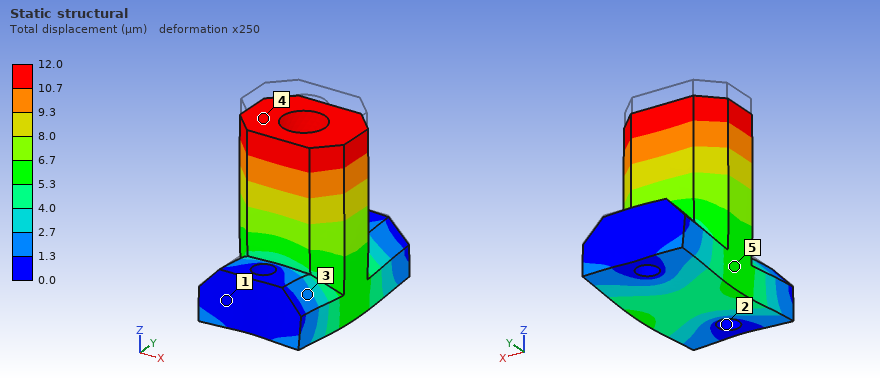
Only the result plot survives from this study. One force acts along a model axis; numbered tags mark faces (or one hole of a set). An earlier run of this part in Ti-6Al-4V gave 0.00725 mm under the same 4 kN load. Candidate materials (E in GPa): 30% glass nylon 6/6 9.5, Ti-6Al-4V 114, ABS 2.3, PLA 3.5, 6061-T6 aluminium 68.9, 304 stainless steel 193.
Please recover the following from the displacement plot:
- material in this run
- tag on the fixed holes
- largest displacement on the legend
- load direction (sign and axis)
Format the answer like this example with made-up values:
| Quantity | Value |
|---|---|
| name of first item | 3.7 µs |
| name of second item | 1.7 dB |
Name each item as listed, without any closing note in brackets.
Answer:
| Quantity | Value |
|---|---|
| material in this run | 6061-T6 aluminium |
| tag on the fixed holes | 2 |
| largest displacement on the legend | 12.0 µm |
| load direction | -Z |
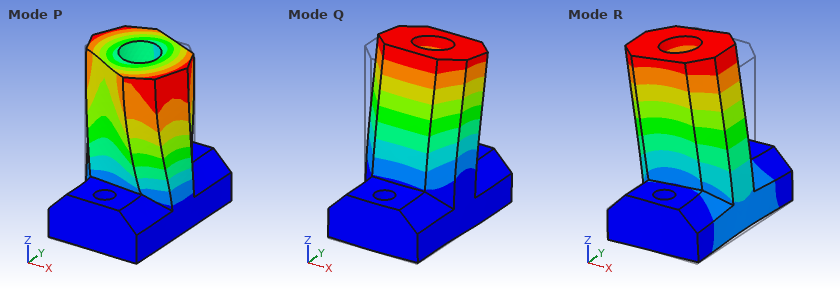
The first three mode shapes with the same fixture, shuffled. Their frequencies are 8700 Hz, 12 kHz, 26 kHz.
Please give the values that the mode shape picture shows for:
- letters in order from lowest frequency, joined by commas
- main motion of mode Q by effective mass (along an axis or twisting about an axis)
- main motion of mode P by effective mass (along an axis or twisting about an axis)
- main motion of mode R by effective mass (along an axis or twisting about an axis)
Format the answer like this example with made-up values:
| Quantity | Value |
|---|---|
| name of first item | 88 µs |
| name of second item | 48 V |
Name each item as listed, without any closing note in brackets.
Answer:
| Quantity | Value |
|---|---|
| letters in order from lowest frequency, joined by commas | R, Q, P |
| main motion of mode Q by effective mass | along Y |
| main motion of mode P by effective mass | twisting about Z |
| main motion of mode R by effective mass | along X |
